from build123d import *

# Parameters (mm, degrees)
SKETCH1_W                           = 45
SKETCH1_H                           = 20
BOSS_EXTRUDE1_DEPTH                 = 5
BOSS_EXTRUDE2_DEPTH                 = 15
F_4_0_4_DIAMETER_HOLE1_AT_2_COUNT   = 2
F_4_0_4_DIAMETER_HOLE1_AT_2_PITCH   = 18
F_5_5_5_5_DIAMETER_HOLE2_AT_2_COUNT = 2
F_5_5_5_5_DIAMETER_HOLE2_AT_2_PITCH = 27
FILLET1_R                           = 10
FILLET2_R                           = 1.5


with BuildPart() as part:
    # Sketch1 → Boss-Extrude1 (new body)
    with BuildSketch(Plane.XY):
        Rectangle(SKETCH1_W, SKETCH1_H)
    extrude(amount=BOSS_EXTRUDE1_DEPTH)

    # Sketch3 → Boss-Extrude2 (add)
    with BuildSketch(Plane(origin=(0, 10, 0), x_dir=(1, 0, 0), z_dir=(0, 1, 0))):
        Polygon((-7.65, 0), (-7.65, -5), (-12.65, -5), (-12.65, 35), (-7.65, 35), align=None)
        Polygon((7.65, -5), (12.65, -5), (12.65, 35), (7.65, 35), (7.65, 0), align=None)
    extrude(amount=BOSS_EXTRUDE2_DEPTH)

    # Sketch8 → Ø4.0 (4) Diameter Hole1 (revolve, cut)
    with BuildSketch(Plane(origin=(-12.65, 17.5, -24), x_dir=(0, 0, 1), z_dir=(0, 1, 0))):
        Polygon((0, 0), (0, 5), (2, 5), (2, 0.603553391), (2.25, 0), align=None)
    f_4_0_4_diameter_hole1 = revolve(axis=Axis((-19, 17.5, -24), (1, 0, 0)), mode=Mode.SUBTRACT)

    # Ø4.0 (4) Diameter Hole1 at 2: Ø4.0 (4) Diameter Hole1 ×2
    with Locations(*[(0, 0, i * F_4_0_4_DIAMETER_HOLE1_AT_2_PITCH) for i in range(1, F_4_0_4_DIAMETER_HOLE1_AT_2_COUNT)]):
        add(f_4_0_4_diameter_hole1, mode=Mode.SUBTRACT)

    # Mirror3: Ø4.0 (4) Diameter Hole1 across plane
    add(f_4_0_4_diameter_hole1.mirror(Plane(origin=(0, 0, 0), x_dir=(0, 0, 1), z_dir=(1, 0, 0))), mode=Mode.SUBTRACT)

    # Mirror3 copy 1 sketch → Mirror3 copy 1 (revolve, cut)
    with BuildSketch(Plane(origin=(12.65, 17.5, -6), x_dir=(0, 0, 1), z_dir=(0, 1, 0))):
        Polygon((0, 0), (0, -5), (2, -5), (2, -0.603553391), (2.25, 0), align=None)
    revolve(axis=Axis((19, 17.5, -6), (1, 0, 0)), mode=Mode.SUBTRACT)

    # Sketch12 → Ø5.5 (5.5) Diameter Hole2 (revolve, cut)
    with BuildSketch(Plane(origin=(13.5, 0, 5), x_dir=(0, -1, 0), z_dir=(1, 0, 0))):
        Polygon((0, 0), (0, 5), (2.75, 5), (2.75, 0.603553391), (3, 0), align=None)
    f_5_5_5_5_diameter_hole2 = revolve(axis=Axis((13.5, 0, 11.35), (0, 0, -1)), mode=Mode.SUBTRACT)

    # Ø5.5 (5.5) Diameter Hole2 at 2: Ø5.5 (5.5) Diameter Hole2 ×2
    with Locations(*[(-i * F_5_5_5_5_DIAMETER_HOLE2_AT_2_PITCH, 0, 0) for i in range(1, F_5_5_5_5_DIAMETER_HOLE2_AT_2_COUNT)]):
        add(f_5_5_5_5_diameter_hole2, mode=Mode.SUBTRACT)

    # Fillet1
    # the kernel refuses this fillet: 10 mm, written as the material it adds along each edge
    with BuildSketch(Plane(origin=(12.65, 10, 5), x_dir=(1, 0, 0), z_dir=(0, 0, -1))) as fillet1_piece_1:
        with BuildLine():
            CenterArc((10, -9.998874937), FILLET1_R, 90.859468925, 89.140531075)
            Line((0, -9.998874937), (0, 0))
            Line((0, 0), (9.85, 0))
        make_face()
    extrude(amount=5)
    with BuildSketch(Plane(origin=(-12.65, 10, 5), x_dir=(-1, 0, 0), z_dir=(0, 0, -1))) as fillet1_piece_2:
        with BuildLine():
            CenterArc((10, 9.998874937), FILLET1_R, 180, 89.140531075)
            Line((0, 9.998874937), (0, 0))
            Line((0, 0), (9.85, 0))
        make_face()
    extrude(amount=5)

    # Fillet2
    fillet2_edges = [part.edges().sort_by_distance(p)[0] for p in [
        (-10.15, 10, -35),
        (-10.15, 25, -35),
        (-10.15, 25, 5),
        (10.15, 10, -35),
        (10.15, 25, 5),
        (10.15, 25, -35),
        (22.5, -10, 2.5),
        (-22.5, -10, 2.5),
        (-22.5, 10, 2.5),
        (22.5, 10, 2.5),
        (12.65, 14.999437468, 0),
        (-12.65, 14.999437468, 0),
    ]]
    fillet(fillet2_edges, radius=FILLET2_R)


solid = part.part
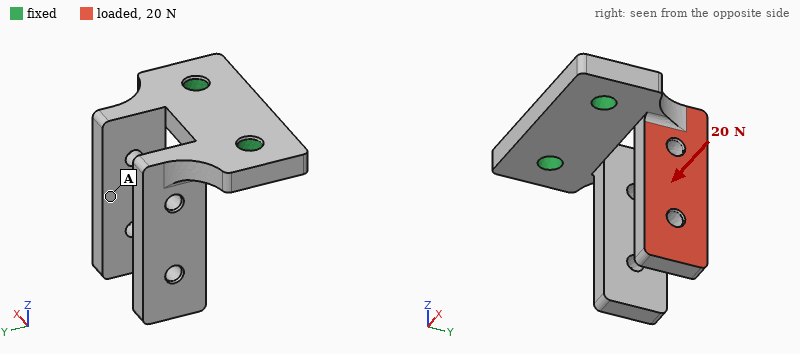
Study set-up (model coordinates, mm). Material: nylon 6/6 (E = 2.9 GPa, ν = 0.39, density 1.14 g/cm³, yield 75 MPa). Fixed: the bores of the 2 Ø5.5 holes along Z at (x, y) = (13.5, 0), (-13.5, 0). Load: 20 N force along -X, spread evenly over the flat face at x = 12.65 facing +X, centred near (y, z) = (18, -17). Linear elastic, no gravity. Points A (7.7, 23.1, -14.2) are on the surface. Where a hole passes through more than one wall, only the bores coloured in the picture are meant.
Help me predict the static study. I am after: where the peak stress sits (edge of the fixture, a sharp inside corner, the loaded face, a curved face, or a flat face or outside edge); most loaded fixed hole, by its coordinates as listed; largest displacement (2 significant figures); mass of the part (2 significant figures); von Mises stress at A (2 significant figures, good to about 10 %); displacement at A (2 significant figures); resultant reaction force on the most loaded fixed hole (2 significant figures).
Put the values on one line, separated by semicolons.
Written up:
a sharp inside corner; (13.5, 0); 0.68 mm; 12 g; 1.9 MPa; 0.27 mm; 18 N
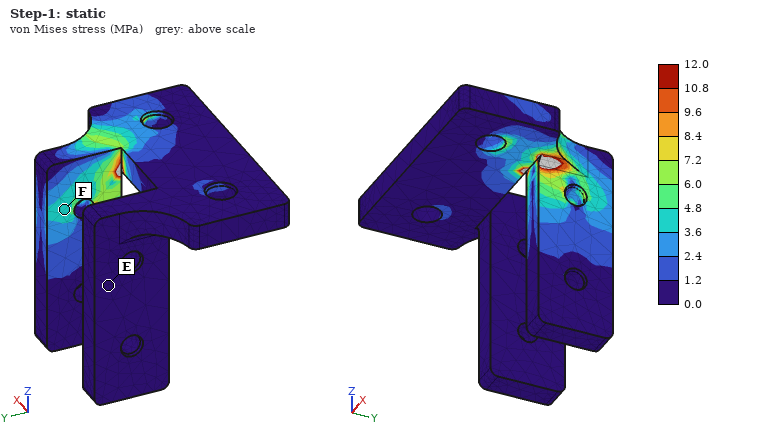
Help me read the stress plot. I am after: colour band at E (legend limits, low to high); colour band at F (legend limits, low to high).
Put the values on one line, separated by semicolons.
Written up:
0.0 to 1.2 MPa; 3.6 to 4.8 MPa
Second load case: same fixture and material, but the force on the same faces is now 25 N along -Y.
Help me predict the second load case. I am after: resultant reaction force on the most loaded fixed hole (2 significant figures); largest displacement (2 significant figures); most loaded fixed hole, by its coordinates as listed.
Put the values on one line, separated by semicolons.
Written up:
24 N; 0.70 mm; (13.5, 0)
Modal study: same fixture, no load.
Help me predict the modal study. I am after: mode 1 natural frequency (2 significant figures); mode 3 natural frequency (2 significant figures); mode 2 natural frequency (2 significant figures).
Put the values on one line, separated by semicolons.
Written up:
600 Hz; 660 Hz; 640 Hz
